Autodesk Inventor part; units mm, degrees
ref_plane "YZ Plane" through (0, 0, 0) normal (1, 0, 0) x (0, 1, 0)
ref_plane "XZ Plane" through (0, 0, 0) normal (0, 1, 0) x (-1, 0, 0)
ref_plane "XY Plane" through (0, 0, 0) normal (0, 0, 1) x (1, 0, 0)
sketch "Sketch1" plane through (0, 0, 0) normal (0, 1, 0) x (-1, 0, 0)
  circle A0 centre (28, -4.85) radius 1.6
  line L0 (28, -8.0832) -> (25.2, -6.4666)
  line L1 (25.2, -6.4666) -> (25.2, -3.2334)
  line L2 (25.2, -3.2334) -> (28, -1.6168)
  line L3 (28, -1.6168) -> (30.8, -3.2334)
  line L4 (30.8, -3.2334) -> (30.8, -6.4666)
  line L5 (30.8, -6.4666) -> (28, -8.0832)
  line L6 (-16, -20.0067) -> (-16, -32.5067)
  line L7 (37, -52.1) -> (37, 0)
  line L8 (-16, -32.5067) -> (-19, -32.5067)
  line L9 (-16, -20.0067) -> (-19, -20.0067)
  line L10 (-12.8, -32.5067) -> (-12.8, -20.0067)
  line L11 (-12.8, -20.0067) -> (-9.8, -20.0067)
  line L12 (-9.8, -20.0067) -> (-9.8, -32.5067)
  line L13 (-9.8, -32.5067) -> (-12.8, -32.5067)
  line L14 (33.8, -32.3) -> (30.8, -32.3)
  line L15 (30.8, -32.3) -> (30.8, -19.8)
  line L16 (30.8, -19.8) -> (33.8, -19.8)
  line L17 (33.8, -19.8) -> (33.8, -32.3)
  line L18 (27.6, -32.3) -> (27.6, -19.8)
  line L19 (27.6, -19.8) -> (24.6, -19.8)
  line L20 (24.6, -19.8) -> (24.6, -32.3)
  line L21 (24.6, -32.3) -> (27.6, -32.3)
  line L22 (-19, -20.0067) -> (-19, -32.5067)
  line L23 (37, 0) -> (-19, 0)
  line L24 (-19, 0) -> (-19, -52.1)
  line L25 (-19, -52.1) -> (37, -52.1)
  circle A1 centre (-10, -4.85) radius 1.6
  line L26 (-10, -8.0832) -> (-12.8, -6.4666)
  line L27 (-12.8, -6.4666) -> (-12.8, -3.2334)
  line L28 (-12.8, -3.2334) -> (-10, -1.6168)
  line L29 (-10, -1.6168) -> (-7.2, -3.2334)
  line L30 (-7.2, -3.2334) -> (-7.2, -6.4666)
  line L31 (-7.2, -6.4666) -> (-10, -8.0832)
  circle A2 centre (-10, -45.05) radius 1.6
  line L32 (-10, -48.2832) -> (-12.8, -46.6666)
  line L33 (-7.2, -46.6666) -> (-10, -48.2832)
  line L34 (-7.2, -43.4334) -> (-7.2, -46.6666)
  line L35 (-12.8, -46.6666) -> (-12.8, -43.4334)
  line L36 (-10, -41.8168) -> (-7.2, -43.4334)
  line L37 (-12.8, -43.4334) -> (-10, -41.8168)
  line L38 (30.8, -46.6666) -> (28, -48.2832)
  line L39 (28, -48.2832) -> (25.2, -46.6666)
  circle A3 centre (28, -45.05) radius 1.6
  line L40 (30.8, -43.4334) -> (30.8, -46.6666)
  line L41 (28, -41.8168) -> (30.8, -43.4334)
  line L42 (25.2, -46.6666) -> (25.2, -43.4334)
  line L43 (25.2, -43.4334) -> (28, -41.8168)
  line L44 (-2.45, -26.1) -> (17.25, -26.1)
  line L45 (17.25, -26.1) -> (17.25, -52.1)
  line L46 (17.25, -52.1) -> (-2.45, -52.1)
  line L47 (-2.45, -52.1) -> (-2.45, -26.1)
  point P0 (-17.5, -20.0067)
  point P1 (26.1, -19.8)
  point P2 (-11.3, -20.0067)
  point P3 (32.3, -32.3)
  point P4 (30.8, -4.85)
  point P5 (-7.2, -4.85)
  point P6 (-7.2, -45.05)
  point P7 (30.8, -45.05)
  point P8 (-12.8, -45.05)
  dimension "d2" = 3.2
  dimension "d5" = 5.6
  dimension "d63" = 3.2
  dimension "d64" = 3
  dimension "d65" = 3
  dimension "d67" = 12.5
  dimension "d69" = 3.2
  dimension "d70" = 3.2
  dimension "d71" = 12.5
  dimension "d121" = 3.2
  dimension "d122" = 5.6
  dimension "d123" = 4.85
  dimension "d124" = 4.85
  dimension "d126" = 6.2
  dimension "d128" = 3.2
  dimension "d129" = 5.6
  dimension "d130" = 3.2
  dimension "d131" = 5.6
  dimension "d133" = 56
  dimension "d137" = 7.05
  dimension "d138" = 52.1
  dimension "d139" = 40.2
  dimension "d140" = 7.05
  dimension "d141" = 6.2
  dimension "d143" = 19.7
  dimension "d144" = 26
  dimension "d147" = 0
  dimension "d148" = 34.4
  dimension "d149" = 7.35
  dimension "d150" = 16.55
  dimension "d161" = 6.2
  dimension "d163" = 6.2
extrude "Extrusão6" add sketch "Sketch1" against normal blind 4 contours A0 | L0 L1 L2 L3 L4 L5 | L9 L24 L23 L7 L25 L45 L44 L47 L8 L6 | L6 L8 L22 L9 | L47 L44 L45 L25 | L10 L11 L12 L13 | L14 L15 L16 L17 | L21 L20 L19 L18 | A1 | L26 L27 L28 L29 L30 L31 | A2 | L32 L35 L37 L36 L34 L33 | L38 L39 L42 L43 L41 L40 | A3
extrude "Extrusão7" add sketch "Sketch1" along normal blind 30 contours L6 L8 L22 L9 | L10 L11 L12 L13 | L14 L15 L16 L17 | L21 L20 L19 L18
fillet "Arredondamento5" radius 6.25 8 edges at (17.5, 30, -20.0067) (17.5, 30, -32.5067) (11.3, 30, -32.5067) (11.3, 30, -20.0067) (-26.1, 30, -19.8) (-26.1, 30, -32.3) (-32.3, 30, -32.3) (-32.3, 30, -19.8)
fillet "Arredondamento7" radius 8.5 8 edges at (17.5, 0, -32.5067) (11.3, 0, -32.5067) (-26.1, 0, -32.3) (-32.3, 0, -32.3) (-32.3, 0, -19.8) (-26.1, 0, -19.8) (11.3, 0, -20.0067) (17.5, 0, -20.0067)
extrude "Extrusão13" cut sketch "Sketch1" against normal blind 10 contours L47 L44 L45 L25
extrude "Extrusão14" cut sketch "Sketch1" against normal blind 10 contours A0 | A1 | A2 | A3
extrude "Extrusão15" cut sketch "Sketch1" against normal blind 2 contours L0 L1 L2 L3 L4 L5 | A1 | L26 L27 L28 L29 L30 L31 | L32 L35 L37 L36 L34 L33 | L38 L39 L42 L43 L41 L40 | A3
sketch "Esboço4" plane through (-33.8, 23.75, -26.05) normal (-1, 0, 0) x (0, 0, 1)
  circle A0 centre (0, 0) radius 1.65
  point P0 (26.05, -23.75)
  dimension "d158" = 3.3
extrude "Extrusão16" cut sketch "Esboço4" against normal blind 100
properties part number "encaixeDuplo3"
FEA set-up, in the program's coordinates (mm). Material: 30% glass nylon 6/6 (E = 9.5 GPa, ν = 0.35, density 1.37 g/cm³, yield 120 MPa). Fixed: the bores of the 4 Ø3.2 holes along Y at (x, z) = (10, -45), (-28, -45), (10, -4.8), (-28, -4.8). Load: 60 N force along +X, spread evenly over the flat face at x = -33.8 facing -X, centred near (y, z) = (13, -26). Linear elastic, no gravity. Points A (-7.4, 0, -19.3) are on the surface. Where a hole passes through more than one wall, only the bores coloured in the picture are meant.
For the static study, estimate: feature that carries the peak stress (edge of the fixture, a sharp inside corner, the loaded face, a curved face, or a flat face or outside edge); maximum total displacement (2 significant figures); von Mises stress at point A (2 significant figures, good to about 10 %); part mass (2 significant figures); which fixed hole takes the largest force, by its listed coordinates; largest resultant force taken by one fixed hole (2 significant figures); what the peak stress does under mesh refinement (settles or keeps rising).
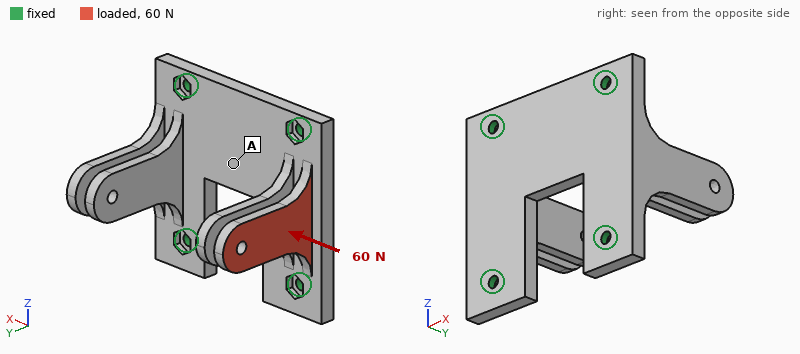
edge of the fixture
0.77 mm
2.5 MPa
19 g
(10, -4.8)
56 N
keeps rising
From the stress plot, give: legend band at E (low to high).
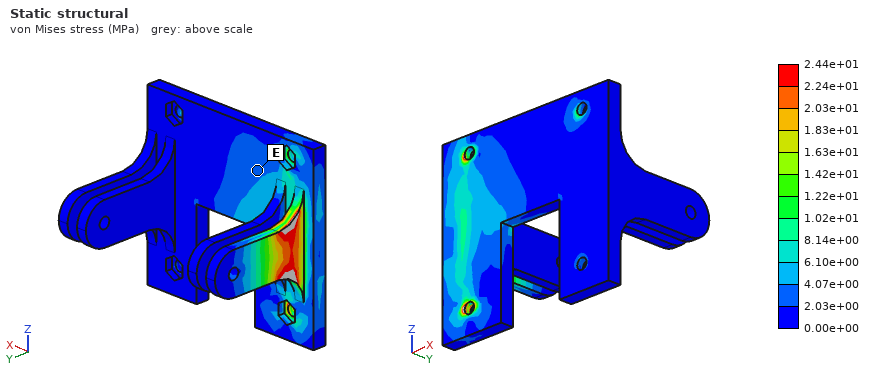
2.03e+00 to 4.07e+00 MPa
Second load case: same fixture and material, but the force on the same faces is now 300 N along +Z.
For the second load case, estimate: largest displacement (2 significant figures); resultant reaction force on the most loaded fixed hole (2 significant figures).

0.31 mm
210 N
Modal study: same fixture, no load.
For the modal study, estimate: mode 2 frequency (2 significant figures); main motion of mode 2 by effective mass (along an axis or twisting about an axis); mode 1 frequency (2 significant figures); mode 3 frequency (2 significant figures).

1400 Hz
along X
1300 Hz
1600 Hz
